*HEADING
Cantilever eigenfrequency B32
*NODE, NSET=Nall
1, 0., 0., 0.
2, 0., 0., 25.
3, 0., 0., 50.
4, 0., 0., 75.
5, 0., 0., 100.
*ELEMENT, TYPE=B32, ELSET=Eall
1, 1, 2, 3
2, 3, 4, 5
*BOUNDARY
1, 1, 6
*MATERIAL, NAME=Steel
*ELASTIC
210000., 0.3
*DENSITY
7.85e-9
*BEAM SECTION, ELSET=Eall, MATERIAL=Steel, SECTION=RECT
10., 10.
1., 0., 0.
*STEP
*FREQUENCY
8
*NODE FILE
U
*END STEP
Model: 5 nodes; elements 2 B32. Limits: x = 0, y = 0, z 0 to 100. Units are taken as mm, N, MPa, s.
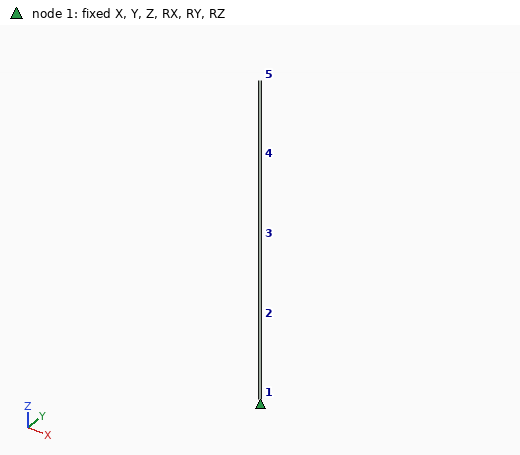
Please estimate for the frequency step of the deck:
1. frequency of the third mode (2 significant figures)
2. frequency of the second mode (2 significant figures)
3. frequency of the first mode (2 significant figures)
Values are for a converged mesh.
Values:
5000 Hz
830 Hz
830 Hz
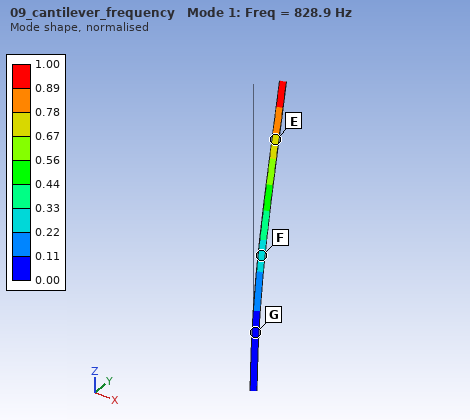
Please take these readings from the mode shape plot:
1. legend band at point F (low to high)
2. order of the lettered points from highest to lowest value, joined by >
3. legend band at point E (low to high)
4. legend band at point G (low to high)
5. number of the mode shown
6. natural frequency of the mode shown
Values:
0.22 to 0.33
E > F > G
0.67 to 0.78
0.00 to 0.11
1
828.9 Hz
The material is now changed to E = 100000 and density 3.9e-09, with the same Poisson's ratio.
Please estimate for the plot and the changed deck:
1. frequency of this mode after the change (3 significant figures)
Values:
812 Hz
